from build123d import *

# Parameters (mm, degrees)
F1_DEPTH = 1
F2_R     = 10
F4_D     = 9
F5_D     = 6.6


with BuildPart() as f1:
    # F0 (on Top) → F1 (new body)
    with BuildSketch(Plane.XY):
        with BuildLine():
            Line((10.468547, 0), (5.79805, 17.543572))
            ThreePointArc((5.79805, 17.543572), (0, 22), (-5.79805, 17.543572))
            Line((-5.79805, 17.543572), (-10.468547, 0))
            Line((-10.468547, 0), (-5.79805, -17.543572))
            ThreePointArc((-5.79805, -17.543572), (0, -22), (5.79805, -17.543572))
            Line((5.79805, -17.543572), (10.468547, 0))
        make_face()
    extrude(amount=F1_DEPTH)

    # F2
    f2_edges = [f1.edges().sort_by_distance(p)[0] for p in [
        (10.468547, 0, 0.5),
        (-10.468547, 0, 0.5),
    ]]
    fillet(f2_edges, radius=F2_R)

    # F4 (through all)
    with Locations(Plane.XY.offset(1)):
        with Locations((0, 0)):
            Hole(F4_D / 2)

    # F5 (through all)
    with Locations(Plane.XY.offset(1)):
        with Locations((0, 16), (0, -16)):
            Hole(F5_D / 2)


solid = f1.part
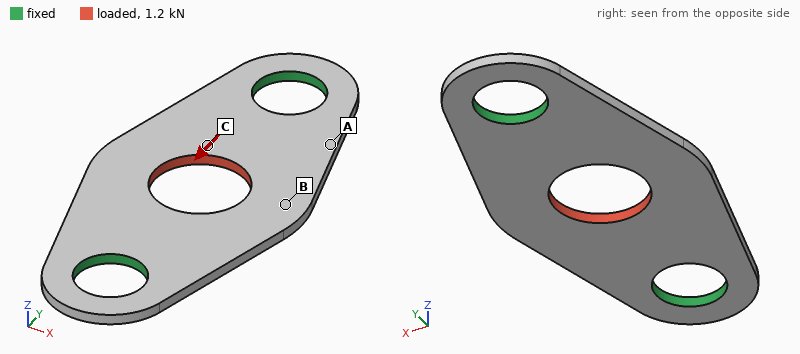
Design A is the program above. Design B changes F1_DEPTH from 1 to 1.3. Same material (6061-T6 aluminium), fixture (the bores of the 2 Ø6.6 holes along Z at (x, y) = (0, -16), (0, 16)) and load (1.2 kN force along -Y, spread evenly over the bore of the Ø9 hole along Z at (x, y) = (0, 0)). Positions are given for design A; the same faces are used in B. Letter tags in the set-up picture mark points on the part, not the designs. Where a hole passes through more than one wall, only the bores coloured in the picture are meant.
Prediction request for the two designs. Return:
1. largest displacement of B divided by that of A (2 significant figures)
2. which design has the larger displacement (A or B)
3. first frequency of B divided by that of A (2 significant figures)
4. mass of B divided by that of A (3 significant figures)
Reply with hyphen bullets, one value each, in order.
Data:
- 0.77
- A
- 1.3
- 1.30
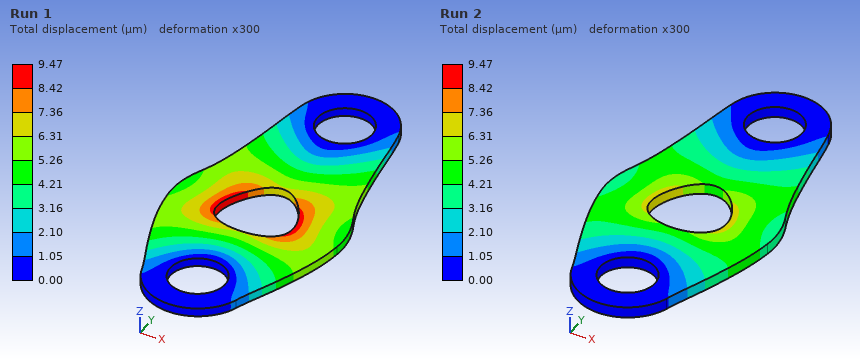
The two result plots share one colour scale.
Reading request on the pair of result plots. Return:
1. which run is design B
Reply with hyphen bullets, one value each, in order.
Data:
- Run 2
